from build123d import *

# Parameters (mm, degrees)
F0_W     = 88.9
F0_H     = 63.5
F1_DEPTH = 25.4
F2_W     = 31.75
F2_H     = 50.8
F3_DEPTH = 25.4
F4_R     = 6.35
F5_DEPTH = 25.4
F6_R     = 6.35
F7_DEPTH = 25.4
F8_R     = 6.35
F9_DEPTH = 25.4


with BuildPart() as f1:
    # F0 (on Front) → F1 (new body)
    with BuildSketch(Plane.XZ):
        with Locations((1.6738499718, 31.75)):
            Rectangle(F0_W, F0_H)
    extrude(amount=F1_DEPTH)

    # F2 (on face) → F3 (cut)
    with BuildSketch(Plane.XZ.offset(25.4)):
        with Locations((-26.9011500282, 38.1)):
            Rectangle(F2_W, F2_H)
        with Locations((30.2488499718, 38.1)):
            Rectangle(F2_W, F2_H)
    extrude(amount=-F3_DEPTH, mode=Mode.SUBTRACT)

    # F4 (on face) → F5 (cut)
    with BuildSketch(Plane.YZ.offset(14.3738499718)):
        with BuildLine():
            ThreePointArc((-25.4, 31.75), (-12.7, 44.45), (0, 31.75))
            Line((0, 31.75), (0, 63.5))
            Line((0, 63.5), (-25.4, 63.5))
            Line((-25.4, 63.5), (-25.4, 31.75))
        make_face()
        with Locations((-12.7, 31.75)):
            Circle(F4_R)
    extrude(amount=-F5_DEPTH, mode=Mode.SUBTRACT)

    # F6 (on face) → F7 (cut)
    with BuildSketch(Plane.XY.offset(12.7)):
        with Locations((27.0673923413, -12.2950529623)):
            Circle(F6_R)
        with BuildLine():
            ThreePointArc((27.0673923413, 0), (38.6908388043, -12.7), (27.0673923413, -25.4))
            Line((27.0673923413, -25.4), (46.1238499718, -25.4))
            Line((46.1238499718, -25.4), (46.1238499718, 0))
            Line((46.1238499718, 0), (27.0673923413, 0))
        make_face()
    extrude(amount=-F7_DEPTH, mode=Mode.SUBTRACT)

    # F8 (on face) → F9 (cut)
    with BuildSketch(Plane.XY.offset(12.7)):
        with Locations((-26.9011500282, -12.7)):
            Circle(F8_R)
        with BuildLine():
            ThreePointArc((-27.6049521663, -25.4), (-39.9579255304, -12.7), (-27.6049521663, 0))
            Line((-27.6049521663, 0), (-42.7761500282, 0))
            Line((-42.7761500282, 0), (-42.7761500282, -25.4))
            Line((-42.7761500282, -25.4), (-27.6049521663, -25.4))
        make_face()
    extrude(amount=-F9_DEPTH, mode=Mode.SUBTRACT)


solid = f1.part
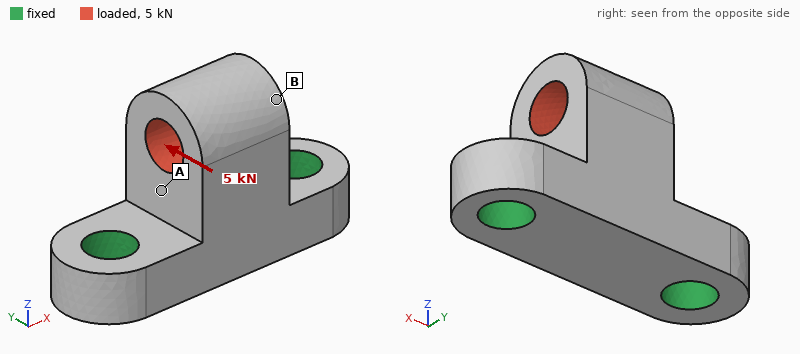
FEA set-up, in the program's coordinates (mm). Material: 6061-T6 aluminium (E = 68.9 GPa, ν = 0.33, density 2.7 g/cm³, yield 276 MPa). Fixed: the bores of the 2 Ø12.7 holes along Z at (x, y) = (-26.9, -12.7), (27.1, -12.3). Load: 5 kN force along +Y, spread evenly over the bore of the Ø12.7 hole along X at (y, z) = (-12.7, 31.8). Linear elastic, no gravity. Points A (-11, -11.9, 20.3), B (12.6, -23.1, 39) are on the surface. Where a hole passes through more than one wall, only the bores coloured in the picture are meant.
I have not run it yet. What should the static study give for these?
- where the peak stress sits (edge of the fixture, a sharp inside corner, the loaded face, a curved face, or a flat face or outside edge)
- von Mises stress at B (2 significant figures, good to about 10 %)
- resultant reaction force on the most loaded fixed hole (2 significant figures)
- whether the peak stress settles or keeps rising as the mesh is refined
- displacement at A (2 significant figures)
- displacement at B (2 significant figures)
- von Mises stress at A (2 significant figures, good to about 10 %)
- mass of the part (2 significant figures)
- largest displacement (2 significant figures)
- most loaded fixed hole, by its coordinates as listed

edge of the fixture
16 MPa
2.8 kN
keeps rising
0.043 mm
0.11 mm
37 MPa
97 g
0.12 mm
(27.1, -12.3)
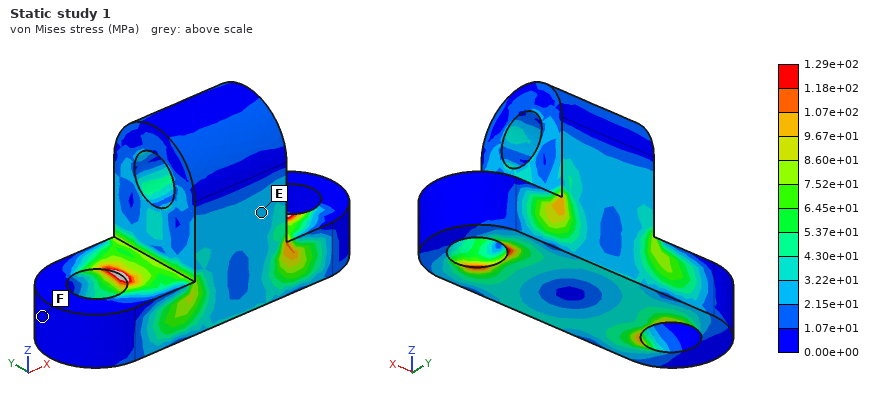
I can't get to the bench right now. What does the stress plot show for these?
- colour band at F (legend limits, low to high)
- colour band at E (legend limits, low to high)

0.00e+00 to 1.07e+01 MPa
2.15e+01 to 3.22e+01 MPa
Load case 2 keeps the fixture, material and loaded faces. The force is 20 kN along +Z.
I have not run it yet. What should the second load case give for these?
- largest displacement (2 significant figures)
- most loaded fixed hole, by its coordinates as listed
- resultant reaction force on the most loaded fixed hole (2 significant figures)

54 µm
(27.1, -12.3)
11 kN
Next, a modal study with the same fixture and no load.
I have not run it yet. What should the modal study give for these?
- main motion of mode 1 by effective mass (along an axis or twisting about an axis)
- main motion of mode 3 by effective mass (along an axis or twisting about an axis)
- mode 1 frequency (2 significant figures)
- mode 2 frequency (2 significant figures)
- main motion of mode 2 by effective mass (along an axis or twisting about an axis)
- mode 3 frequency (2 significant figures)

along Y
along Z
6600 Hz
12 kHz
along X
16 kHz
